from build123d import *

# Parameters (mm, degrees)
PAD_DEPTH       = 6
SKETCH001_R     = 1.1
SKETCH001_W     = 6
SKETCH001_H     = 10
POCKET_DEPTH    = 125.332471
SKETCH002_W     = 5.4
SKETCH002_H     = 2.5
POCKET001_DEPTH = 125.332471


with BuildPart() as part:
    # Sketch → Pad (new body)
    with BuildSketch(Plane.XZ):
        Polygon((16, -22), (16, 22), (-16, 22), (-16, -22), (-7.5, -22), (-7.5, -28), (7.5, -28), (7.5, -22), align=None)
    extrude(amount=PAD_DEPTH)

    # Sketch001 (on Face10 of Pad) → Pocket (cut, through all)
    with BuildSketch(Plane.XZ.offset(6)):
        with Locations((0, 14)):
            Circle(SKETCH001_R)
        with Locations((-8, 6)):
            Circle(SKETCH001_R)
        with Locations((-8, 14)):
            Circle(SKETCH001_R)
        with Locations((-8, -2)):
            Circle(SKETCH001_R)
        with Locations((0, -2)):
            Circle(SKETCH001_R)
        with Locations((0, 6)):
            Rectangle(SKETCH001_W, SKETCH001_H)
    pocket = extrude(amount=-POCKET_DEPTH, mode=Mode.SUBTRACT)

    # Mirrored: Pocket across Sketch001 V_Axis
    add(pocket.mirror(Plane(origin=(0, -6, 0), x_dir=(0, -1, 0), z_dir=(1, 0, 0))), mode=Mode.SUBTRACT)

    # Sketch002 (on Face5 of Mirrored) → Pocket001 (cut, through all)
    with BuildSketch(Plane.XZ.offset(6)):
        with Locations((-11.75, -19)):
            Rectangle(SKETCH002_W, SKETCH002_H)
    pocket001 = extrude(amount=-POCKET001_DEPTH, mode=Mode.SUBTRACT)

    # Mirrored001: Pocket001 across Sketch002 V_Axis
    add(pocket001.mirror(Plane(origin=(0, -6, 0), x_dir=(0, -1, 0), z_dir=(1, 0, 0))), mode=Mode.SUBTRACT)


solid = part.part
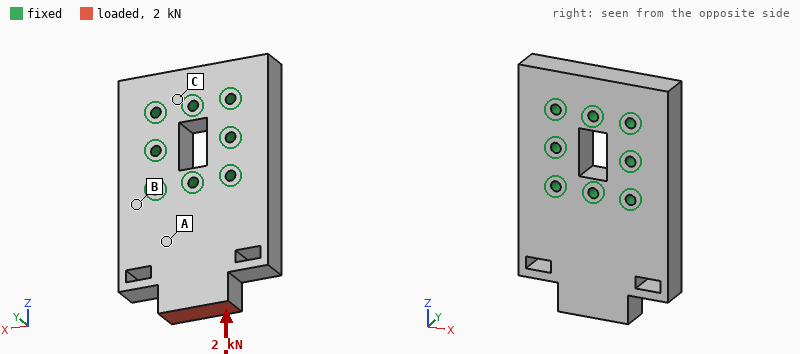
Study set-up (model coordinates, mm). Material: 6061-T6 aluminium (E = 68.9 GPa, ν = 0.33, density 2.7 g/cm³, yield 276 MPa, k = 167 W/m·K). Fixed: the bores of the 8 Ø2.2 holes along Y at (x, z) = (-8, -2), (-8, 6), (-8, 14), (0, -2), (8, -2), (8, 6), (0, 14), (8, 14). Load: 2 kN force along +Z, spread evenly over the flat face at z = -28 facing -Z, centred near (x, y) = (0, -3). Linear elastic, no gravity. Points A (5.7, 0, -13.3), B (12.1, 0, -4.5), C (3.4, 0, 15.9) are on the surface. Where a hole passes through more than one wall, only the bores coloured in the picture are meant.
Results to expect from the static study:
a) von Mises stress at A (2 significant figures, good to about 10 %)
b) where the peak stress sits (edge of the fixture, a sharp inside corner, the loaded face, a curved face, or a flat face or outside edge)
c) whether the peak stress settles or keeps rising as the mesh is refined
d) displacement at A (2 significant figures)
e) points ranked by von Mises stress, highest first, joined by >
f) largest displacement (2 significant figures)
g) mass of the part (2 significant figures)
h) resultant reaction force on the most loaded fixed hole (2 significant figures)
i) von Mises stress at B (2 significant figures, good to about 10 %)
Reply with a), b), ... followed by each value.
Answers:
a) 16 MPa
b) edge of the fixture
c) keeps rising
d) 2.4 µm
e) A > B > C
f) 6.6 µm
g) 22 g
h) 590 N
i) 5.9 MPa
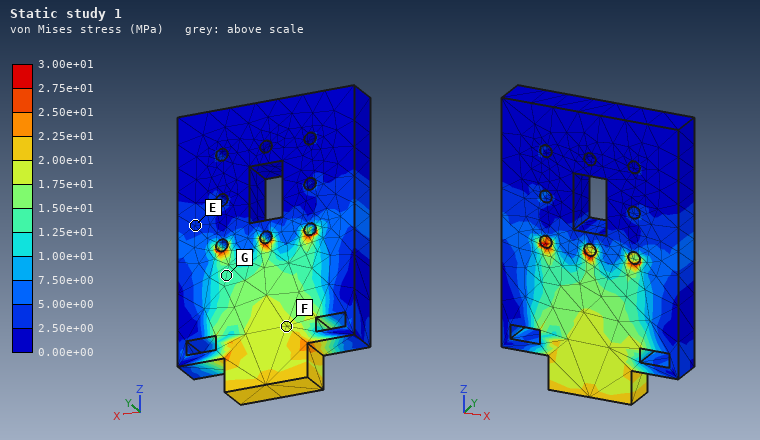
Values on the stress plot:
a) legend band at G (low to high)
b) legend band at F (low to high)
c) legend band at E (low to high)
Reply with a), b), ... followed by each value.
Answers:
a) 1.25e+01 to 1.50e+01 MPa
b) 1.75e+01 to 2.00e+01 MPa
c) 2.50e+00 to 5.00e+00 MPa
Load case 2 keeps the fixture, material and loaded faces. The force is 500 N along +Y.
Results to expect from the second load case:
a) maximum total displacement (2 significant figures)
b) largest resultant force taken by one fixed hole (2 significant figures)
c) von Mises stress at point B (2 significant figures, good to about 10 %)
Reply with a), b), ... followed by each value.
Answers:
a) 93 µm
b) 290 N
c) 41 MPa
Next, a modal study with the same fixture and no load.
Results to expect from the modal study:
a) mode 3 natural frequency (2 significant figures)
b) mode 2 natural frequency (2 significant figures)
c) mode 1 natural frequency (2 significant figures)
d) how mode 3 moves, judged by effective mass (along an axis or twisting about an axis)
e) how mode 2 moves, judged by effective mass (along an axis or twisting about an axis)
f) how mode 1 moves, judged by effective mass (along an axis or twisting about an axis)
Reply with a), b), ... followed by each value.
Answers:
a) 23 kHz
b) 17 kHz
c) 8500 Hz
d) along X
e) twisting about Z
f) along Y
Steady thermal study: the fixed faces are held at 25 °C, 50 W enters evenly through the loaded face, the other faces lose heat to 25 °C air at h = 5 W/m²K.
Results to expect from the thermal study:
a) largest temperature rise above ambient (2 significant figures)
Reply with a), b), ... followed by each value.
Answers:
a) 61 K
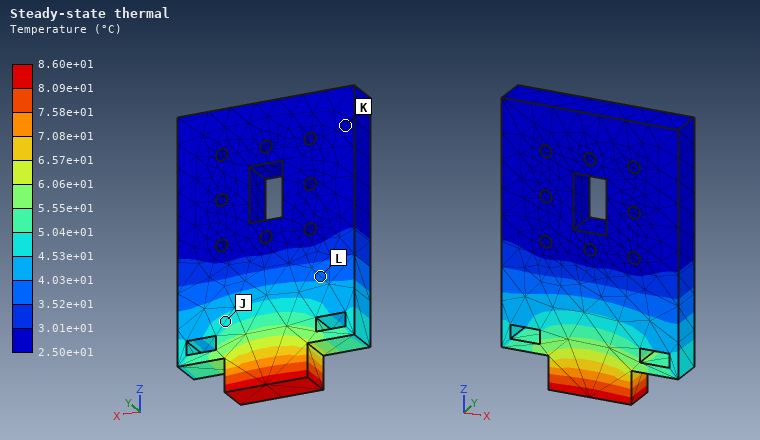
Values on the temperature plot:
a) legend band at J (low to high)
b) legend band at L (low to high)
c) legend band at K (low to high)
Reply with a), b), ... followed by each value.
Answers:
a) 4.53e+01 to 5.04e+01 °C
b) 3.52e+01 to 4.03e+01 °C
c) 2.50e+01 to 3.01e+01 °C
